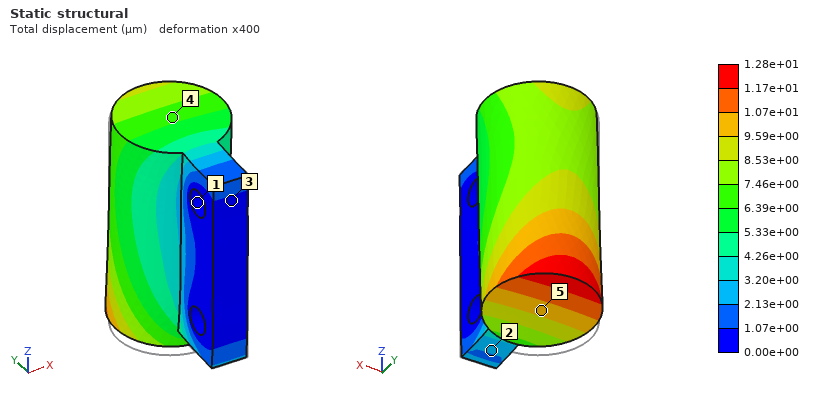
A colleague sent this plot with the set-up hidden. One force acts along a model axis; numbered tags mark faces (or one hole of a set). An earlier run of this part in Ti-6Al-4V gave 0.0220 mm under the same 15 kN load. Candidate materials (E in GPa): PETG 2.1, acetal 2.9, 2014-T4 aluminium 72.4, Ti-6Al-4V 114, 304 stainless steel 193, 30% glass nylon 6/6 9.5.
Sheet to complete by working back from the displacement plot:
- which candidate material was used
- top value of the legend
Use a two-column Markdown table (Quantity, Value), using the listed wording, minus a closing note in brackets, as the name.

| Quantity | Value |
|---|---|
| which candidate material was used | 304 stainless steel |
| top value of the legend | 1.28e+01 µm |
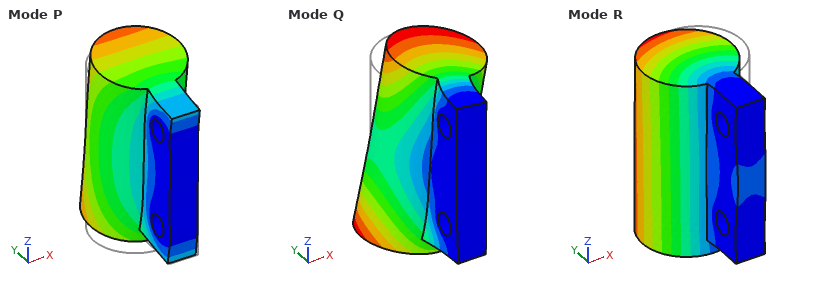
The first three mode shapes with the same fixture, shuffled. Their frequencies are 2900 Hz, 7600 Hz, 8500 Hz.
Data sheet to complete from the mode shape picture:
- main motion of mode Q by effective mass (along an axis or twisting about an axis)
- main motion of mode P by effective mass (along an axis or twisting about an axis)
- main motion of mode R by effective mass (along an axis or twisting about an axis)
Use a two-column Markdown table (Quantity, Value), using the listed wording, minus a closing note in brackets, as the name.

| Quantity | Value |
|---|---|
| main motion of mode Q by effective mass | twisting about Y |
| main motion of mode P by effective mass | along Z |
| main motion of mode R by effective mass | along X |
